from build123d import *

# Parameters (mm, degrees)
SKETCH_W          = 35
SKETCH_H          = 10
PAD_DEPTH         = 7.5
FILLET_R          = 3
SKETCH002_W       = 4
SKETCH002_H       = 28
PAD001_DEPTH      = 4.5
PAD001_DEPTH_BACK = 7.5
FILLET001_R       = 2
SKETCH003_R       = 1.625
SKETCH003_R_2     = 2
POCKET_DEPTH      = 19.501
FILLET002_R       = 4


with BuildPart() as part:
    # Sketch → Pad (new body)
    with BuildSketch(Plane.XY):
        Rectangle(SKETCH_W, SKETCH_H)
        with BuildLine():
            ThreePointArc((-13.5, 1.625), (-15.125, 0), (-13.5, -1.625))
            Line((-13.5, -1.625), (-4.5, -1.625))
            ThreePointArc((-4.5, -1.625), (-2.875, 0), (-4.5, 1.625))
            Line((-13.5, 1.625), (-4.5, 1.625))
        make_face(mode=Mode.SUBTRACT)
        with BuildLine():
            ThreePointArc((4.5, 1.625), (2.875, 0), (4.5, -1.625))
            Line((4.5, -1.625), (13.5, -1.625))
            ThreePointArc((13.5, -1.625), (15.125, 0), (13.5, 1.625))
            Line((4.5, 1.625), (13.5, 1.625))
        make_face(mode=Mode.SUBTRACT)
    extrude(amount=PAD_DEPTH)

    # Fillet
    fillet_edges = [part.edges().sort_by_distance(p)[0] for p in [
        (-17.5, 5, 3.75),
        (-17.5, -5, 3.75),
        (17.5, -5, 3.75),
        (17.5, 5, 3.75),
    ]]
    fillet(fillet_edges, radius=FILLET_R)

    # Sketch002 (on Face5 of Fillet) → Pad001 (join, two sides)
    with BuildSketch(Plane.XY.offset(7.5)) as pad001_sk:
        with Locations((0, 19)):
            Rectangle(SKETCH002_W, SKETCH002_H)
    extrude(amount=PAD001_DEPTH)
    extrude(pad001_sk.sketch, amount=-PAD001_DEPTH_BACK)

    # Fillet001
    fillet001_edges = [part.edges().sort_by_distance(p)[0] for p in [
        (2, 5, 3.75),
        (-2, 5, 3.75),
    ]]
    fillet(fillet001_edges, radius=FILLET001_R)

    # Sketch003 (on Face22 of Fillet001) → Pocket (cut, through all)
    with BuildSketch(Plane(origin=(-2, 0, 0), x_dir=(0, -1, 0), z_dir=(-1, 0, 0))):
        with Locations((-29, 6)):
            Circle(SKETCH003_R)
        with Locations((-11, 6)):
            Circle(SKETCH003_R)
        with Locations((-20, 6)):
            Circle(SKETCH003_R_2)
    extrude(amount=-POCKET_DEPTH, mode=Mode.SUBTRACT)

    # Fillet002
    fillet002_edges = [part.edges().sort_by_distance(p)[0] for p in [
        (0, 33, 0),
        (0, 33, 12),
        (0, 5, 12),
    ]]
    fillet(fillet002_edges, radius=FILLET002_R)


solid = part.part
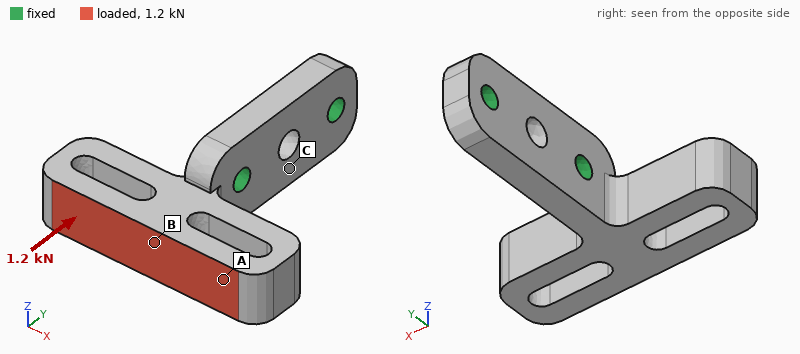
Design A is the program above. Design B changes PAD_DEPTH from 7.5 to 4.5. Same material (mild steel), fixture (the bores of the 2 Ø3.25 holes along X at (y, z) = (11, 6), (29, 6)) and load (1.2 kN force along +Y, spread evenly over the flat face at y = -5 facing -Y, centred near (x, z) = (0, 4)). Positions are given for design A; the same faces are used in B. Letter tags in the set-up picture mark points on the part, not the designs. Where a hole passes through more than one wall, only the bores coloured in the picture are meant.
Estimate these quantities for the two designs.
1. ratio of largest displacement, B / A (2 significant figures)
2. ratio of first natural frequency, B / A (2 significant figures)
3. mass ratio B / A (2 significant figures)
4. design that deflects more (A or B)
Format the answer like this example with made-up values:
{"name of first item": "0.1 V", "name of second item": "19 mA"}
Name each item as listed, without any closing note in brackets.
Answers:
{"ratio of largest displacement, B / A": "1.7", "ratio of first natural frequency, B / A": "1.1", "mass ratio B / A": "0.75", "design that deflects more": "B"}
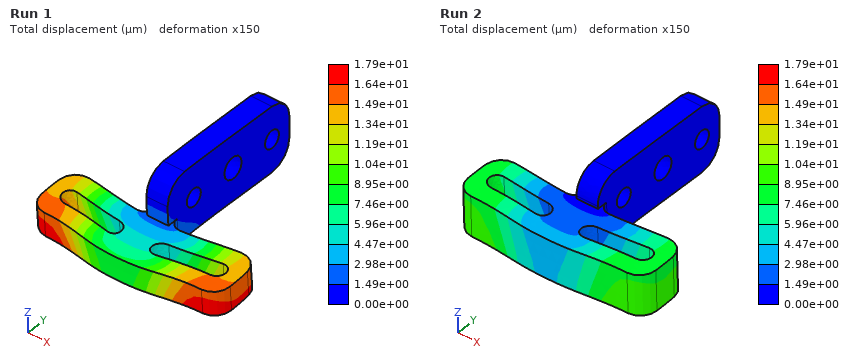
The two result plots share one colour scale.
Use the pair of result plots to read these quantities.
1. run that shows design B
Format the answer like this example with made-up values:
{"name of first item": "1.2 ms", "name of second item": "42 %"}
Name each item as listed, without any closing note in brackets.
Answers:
{"run that shows design B": "Run 1"}
